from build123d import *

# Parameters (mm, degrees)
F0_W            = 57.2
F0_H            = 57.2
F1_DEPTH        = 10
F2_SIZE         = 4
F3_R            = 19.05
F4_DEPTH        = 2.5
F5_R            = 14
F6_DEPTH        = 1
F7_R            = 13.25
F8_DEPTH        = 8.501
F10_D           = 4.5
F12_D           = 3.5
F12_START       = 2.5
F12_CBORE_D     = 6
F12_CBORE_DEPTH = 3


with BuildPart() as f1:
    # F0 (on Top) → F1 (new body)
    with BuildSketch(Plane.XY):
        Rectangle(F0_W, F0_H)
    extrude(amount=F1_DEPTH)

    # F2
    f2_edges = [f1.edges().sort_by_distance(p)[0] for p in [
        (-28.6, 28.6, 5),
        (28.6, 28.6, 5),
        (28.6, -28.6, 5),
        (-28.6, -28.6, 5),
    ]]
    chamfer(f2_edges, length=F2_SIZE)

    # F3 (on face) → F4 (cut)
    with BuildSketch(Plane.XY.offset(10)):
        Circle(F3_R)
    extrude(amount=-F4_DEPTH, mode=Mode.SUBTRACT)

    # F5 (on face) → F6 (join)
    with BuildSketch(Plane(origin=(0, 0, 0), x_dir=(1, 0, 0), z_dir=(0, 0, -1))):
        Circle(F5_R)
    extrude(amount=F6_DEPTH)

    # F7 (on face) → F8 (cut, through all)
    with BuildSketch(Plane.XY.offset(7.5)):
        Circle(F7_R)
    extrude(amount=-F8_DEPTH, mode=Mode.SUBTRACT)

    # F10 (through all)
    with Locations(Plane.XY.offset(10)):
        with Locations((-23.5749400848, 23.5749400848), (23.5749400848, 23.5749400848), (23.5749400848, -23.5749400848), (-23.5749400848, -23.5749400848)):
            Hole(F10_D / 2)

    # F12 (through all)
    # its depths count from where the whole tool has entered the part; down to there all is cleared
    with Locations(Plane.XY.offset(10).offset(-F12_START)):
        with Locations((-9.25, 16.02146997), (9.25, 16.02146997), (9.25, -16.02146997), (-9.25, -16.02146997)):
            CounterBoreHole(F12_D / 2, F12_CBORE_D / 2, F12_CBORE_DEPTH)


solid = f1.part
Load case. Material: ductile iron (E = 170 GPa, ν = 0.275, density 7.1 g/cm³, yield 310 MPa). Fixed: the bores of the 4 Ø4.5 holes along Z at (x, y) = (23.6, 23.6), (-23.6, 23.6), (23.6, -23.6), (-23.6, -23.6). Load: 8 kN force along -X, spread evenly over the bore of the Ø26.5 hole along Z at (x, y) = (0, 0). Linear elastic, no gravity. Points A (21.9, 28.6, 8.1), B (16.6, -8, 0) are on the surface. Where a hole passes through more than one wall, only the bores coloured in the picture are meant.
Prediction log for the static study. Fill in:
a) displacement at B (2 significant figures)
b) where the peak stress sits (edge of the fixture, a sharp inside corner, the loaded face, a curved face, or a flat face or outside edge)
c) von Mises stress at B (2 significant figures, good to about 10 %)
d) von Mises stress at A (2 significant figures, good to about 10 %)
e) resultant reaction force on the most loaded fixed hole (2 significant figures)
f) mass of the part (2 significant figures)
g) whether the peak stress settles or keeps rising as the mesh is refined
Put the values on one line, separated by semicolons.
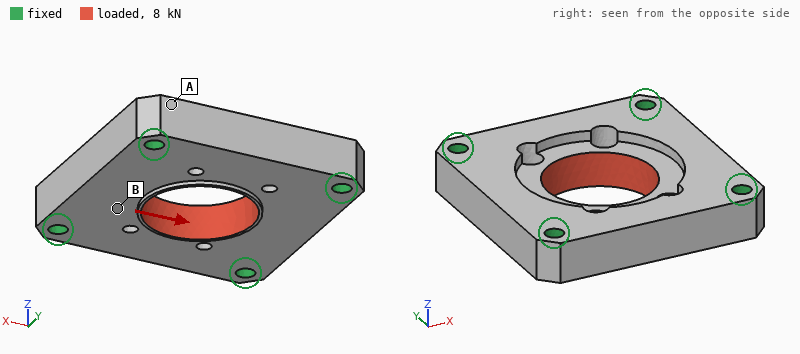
3.3 µm; edge of the fixture; 20 MPa; 5.3 MPa; 2.2 kN; 170 g; keeps rising
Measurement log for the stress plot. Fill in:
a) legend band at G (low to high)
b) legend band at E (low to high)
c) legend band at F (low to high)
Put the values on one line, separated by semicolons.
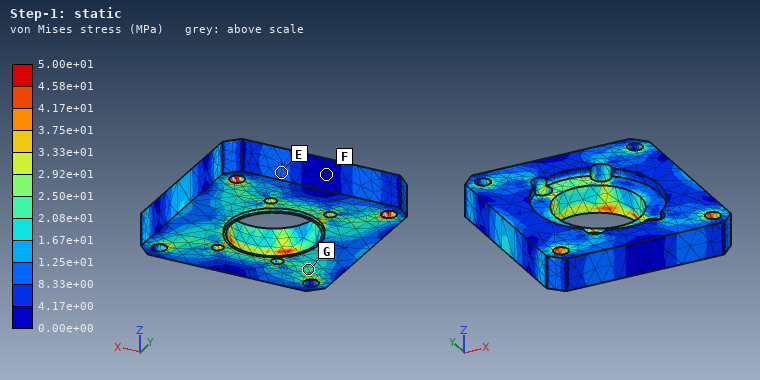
2.08e+01 to 2.50e+01 MPa; 8.33e+00 to 1.25e+01 MPa; 0.00e+00 to 4.17e+00 MPa
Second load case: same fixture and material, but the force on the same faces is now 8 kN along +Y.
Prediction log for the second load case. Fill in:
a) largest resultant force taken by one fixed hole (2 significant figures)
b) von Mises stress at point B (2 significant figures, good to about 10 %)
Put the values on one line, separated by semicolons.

2.2 kN; 16 MPa
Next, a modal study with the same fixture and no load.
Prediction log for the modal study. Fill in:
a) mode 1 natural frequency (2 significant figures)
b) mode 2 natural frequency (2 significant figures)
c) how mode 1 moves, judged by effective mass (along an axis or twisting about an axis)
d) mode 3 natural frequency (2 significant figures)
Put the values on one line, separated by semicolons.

15 kHz; 18 kHz; along Z; 18 kHz
